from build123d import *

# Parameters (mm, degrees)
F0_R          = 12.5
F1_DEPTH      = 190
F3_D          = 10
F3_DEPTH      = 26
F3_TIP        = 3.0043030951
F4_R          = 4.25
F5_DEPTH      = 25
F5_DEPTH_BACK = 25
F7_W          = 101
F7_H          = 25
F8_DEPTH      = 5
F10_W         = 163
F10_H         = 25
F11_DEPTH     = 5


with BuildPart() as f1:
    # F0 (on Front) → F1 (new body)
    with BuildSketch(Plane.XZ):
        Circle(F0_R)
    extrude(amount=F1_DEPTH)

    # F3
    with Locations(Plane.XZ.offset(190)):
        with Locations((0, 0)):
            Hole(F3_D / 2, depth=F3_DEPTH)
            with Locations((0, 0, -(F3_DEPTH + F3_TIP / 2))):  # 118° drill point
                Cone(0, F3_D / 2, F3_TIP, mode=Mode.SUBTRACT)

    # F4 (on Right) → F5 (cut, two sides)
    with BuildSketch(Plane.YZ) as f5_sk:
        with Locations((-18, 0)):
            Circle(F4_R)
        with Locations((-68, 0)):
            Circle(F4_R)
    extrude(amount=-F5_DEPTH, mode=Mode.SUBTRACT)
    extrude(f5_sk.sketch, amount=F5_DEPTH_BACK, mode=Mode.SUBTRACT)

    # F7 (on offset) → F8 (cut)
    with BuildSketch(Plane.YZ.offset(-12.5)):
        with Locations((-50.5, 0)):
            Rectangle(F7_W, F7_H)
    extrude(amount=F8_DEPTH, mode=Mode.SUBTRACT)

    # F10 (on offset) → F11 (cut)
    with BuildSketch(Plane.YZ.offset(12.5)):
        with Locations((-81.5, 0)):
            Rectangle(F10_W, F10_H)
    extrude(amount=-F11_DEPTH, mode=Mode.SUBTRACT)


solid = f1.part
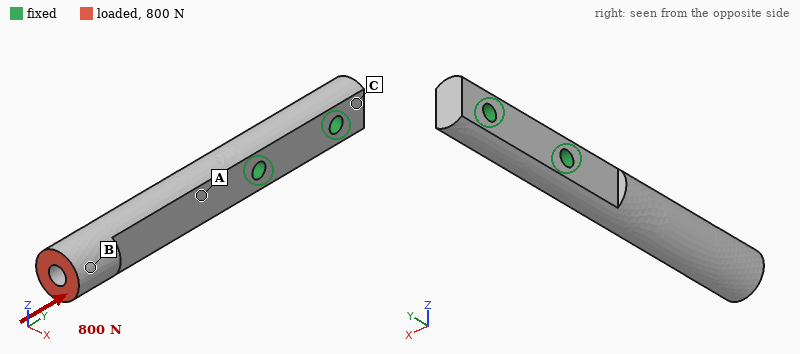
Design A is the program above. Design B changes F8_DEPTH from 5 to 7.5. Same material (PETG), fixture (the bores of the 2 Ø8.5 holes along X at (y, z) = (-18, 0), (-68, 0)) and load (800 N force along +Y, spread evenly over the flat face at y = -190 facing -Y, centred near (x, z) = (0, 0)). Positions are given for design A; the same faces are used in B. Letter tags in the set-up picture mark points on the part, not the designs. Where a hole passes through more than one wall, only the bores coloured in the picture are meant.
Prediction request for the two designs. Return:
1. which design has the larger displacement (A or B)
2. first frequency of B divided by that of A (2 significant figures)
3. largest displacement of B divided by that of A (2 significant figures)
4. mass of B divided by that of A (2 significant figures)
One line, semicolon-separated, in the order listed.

B; 0.80; 1.1; 0.93
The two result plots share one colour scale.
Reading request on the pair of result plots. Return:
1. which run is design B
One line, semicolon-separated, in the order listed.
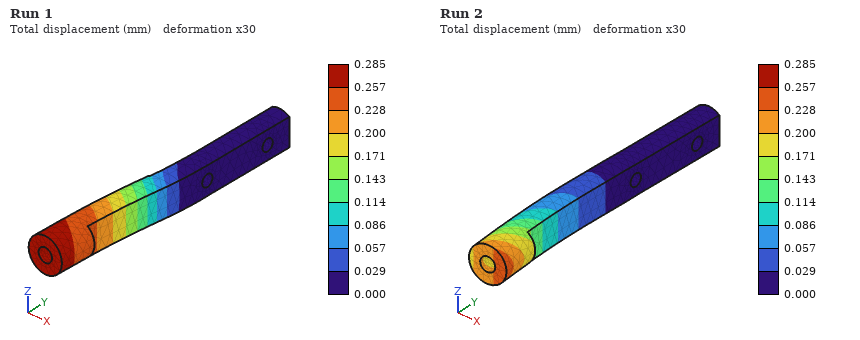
Run 1
